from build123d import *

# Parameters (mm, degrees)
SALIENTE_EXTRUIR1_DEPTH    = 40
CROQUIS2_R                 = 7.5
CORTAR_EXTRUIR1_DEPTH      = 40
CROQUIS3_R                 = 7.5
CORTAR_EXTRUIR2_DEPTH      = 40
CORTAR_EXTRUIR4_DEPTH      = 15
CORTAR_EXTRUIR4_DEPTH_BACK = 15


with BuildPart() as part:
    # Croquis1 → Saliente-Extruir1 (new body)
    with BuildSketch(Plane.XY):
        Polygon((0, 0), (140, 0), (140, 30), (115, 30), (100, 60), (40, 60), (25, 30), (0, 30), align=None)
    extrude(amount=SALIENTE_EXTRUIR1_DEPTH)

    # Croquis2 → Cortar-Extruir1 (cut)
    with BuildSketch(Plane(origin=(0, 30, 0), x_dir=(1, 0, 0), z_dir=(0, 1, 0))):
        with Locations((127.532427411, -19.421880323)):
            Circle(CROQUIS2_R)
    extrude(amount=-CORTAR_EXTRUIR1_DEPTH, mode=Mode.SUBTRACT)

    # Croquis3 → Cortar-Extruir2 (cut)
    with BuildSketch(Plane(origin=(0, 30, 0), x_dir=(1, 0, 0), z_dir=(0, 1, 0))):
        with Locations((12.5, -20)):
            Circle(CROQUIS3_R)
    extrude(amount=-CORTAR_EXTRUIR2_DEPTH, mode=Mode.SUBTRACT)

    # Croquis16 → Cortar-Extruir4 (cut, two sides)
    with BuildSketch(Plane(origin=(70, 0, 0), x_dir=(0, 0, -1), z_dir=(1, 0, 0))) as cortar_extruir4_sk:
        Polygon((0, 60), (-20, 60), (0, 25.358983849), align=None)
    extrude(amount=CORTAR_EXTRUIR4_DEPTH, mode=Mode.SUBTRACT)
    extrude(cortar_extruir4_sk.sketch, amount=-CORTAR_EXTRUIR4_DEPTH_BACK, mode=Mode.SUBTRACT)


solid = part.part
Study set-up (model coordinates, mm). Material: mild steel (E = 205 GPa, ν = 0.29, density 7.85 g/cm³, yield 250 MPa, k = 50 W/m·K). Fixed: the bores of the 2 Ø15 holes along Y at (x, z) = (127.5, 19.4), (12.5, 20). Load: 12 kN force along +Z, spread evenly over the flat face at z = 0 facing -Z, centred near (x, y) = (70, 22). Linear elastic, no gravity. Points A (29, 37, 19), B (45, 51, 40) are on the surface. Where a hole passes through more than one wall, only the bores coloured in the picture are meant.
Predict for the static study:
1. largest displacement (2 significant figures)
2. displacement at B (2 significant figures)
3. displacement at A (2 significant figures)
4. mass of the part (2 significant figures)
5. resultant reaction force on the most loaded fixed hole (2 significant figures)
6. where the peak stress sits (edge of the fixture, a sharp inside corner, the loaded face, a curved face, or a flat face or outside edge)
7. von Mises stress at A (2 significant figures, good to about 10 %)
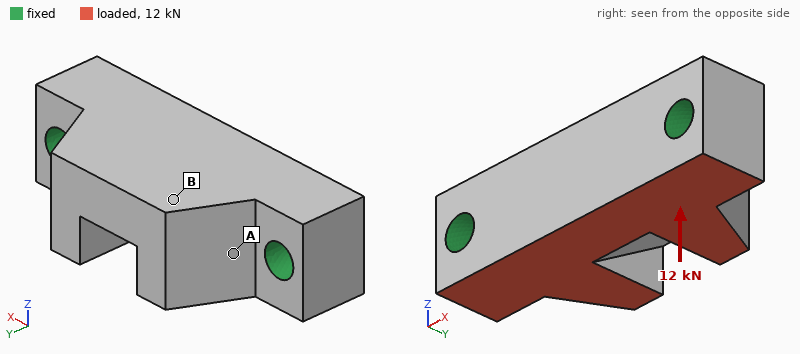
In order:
5.6 µm
4.5 µm
2.5 µm
1.9 kg
6.0 kN
edge of the fixture
8.0 MPa
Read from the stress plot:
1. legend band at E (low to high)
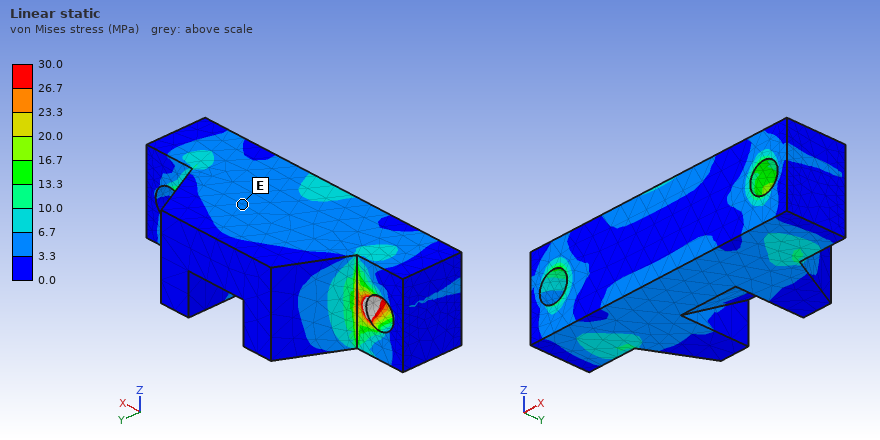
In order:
3.3 to 6.7 MPa
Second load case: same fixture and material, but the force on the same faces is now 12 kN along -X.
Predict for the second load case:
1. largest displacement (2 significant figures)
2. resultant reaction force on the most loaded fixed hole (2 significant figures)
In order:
2.2 µm
6.3 kN
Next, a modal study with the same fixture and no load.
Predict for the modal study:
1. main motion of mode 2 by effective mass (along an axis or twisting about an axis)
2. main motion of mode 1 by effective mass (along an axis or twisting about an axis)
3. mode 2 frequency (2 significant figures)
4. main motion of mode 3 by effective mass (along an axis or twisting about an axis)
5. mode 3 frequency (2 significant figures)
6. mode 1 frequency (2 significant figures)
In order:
along Y
along Z
9200 Hz
along Z
10000 Hz
5800 Hz
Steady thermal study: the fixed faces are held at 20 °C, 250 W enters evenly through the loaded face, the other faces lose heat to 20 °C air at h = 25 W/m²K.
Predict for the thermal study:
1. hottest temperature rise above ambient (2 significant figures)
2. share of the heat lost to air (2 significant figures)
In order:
53 K
5.6 %
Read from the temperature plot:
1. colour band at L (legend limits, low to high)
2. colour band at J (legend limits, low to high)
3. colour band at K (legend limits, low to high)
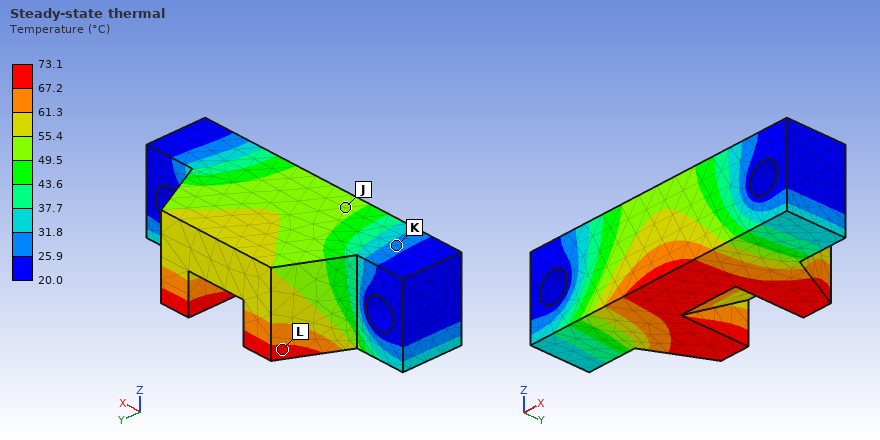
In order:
67.2 to 73.1 °C
49.5 to 55.4 °C
25.9 to 31.8 °C
